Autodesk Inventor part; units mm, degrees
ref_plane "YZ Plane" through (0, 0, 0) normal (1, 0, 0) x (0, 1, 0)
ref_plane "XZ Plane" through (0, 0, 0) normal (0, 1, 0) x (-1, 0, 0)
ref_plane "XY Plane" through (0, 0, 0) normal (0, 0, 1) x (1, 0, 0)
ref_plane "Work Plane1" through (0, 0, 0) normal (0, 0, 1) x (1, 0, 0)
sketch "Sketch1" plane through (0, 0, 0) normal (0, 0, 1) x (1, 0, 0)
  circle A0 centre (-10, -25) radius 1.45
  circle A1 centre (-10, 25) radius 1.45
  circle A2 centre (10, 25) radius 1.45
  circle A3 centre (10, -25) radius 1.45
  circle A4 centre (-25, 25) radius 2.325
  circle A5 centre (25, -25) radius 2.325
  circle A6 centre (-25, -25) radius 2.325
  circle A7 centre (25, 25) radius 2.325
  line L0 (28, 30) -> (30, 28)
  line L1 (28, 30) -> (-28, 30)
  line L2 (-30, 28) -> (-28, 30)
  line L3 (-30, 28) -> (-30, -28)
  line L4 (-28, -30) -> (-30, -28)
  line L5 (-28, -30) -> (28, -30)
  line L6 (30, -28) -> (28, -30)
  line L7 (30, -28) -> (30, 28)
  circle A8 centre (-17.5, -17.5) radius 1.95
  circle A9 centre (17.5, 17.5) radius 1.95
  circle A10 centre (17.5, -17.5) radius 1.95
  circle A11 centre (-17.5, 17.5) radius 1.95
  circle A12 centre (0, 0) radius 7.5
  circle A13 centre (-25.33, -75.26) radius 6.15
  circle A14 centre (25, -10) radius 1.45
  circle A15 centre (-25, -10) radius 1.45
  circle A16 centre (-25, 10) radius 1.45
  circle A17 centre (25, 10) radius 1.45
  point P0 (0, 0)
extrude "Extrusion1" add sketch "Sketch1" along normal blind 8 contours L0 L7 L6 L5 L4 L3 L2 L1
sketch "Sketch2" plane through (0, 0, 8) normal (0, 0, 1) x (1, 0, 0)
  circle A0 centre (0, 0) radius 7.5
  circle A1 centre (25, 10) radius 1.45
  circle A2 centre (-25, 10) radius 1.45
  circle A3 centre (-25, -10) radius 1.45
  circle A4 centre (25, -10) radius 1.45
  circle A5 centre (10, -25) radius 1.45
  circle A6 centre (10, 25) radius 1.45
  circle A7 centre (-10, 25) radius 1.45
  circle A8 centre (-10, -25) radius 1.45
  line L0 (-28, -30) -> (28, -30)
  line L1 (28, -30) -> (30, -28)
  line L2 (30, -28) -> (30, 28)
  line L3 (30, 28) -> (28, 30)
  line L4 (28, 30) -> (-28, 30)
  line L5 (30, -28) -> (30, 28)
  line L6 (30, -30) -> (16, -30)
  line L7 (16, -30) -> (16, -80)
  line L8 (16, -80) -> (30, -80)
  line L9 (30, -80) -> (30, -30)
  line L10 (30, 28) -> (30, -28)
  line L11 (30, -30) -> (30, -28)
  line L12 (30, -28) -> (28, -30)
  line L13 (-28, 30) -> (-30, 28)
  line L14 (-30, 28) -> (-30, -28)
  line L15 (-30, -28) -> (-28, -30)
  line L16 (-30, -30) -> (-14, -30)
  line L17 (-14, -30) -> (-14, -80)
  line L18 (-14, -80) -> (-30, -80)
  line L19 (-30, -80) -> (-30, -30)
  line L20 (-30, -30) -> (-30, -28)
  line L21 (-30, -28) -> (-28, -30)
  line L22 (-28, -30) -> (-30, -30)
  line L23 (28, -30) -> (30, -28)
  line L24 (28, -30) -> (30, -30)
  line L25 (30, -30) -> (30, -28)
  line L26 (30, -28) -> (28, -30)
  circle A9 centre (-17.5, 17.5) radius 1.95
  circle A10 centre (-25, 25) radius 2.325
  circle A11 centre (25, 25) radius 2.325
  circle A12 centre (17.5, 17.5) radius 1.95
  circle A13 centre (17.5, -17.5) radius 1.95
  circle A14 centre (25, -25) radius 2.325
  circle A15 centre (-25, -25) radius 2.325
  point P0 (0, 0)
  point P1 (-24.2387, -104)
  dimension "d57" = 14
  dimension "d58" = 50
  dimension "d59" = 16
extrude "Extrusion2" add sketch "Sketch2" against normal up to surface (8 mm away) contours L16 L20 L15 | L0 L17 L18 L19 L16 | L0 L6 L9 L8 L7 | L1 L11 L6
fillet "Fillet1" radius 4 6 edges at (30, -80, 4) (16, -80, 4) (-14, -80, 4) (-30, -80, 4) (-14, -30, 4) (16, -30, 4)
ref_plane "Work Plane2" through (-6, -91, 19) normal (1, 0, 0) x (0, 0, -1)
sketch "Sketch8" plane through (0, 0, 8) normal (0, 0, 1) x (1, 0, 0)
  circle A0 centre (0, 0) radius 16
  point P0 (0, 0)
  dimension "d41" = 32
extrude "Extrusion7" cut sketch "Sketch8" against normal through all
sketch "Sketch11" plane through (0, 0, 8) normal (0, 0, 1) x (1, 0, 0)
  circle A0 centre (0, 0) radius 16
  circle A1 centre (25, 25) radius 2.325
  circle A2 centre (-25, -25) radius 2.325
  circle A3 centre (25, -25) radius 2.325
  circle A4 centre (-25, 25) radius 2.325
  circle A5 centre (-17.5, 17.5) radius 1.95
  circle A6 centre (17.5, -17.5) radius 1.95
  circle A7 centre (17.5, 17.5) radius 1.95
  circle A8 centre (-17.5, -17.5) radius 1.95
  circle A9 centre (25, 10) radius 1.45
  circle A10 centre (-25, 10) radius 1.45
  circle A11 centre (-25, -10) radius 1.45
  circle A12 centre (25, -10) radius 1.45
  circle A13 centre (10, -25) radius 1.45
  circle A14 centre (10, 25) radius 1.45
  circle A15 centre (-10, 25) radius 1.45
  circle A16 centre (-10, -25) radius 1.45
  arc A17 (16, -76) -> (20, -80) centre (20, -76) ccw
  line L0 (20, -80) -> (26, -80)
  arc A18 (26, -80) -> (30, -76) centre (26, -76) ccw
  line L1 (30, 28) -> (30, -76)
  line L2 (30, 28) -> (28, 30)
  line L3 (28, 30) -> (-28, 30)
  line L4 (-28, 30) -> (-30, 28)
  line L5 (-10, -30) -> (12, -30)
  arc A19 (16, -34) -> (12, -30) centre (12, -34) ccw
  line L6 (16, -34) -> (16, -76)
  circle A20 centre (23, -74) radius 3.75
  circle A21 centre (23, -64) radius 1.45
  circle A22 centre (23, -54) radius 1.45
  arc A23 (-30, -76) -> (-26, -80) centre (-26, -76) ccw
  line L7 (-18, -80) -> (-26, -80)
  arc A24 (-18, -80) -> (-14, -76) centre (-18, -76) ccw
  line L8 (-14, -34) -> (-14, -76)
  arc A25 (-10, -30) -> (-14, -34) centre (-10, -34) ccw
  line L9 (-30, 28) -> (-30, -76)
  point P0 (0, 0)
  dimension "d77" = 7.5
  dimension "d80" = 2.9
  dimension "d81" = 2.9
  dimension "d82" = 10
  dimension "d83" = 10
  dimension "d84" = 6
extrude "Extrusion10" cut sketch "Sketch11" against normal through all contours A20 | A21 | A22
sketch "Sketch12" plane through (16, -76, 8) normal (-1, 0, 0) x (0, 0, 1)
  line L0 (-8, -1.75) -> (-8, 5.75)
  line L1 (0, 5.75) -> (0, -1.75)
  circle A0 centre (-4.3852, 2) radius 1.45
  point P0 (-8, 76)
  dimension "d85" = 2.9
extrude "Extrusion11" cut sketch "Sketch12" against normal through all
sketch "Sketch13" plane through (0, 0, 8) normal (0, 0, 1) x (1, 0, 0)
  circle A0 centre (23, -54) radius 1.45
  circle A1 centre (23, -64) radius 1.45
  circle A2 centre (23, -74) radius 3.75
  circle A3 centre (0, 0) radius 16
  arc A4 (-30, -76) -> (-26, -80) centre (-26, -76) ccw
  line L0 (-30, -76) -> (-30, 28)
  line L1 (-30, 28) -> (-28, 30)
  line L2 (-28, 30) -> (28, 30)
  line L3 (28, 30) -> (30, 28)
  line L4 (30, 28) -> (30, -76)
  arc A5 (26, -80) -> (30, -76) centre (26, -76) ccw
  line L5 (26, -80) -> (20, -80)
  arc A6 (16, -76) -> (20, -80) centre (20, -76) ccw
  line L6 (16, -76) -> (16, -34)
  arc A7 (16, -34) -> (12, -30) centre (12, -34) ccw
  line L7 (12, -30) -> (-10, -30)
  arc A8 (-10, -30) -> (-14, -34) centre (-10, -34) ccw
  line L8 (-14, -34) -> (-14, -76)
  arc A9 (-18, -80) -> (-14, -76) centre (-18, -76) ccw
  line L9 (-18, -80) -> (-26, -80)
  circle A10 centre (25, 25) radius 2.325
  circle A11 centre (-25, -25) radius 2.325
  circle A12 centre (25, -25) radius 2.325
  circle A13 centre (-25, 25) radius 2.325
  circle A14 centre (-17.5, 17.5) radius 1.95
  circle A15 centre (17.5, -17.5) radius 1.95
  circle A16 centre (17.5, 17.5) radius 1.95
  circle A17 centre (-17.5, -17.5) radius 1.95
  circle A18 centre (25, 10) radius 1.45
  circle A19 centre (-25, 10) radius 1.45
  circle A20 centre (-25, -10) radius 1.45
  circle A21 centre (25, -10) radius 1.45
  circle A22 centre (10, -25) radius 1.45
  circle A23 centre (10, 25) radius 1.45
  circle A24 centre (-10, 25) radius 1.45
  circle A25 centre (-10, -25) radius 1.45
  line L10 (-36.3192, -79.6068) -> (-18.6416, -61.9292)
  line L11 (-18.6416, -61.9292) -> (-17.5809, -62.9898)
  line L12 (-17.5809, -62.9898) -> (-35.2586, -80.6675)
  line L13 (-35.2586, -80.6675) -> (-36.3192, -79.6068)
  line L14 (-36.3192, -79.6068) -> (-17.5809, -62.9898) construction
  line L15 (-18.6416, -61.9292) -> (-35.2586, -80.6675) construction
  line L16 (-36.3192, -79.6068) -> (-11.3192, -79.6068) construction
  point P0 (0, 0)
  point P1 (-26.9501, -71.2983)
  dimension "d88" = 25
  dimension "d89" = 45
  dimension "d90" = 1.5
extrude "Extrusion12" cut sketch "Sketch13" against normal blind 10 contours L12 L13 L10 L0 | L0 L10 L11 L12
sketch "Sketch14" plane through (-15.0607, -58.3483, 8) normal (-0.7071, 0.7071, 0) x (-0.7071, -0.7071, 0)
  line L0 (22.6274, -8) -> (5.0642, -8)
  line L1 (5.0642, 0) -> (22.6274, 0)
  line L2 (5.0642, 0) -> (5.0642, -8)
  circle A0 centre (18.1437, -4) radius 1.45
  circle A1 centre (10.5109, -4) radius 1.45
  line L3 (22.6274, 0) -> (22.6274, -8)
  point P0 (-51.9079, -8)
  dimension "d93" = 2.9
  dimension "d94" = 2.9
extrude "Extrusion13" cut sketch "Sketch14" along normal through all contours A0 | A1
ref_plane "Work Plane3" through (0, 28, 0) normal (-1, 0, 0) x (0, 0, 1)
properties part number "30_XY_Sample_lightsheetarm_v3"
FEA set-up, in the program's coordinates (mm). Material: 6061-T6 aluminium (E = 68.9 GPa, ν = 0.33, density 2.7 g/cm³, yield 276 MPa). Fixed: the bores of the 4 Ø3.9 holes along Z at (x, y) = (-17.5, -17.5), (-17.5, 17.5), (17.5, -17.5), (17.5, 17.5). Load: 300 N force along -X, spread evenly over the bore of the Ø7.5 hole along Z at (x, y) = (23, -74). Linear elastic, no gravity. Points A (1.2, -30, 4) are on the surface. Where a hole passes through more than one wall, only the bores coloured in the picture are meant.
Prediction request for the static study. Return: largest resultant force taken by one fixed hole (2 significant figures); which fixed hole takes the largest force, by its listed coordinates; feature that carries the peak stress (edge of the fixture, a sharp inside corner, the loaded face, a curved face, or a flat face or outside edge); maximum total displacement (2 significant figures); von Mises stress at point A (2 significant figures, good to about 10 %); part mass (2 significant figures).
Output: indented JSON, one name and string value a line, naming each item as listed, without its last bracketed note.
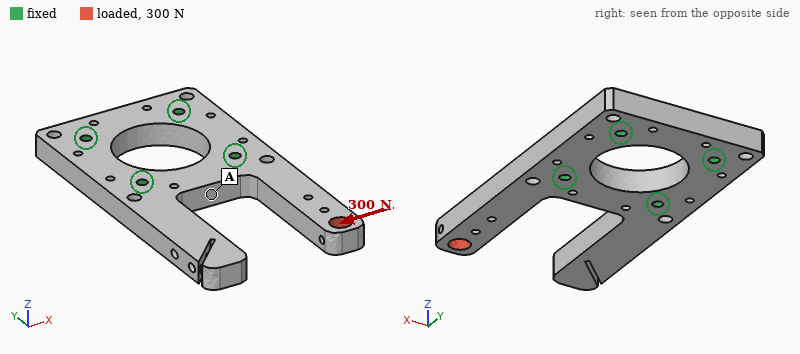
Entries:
{
  "largest resultant force taken by one fixed hole": "480 N",
  "which fixed hole takes the largest force, by its listed coordinates": "(-17.5, -17.5)",
  "feature that carries the peak stress": "a curved face",
  "maximum total displacement": "0.14 mm",
  "von Mises stress at point A": "8.7 MPa",
  "part mass": "87 g"
}
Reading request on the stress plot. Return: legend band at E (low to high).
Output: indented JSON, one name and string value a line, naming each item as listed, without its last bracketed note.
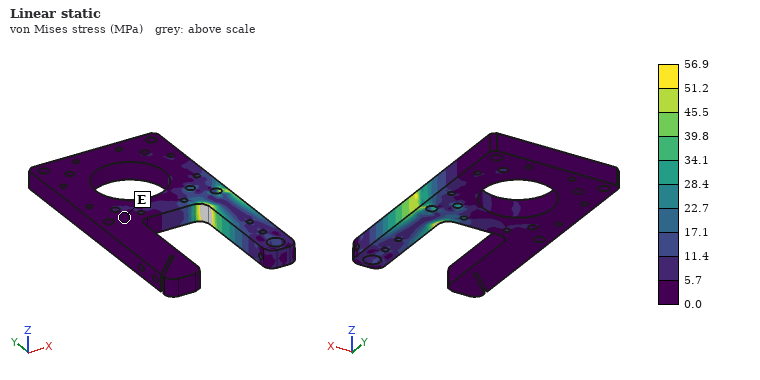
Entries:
{
  "legend band at E": "0.0 to 5.7 MPa"
}
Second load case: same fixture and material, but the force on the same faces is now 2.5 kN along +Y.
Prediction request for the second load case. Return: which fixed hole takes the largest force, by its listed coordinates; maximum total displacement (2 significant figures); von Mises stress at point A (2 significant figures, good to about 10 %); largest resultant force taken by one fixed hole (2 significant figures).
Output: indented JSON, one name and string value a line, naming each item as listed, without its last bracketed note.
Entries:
{
  "which fixed hole takes the largest force, by its listed coordinates": "(17.5, -17.5)",
  "maximum total displacement": "48 µm",
  "von Mises stress at point A": "5.9 MPa",
  "largest resultant force taken by one fixed hole": "2.2 kN"
}
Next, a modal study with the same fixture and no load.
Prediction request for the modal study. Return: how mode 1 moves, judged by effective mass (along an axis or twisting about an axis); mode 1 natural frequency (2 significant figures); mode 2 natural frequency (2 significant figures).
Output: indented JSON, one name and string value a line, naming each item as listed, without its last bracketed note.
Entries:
{
  "how mode 1 moves, judged by effective mass": "along Z",
  "mode 1 natural frequency": "1700 Hz",
  "mode 2 natural frequency": "1900 Hz"
}
